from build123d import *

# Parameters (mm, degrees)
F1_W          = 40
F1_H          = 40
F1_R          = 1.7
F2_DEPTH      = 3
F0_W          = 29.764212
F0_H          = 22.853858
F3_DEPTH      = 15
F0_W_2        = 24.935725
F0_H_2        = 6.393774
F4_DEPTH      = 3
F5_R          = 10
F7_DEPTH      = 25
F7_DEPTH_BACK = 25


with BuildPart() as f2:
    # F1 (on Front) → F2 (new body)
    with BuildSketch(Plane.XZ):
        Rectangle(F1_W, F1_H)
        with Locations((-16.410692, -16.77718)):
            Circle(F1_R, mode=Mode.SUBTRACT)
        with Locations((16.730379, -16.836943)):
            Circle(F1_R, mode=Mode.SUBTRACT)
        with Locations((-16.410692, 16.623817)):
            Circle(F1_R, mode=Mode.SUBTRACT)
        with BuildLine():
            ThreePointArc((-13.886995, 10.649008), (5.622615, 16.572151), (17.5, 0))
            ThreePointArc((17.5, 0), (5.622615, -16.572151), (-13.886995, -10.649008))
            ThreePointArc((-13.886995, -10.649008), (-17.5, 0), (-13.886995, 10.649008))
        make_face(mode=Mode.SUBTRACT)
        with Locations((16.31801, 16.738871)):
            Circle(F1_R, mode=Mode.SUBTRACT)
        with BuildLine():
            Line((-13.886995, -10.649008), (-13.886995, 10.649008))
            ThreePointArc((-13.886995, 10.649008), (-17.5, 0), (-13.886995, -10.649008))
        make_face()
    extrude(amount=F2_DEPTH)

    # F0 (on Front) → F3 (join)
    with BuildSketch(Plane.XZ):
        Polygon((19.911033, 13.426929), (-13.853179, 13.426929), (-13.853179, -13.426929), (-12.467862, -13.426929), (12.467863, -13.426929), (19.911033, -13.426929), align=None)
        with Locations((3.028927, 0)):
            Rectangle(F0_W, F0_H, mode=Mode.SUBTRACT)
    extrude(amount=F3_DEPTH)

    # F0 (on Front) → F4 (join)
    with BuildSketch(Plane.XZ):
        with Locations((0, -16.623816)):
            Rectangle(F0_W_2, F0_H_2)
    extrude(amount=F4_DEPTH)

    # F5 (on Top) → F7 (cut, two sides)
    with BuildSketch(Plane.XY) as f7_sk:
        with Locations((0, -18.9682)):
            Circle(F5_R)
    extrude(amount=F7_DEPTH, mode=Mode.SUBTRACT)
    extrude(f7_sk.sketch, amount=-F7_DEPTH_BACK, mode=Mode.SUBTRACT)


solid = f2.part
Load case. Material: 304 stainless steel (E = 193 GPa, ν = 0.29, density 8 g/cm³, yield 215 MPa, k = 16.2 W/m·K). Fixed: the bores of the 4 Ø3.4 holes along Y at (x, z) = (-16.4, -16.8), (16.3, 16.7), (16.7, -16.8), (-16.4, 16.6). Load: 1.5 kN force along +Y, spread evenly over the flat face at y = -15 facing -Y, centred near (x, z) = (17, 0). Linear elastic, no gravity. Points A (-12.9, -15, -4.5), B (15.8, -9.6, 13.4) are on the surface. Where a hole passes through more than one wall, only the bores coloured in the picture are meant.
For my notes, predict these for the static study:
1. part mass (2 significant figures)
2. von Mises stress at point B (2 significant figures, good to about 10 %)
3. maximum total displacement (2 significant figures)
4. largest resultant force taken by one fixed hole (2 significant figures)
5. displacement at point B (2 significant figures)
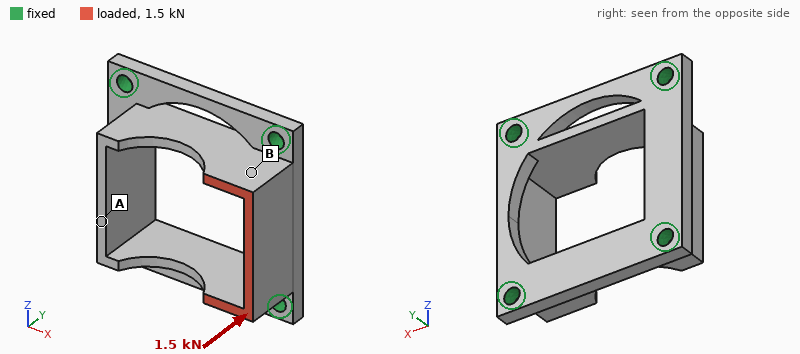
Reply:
40 g
23 MPa
8.6 µm
800 N
4.3 µm
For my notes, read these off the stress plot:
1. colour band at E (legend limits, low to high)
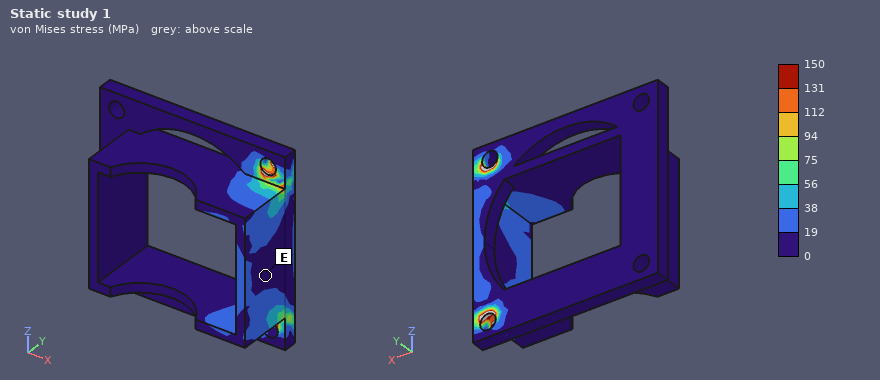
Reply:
0 to 19 MPa
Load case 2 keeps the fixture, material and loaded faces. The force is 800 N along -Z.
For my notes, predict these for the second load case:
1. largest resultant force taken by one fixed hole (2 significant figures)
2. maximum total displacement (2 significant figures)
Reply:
550 N
22 µm
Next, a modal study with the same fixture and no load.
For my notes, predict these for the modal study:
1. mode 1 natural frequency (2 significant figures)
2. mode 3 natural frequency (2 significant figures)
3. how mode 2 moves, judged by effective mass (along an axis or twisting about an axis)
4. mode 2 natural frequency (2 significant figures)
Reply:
11 kHz
14 kHz
along X
13 kHz
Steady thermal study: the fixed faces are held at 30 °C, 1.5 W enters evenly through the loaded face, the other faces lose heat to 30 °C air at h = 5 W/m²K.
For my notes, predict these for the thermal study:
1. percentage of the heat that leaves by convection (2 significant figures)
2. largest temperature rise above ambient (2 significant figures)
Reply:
7.7 %
20 K
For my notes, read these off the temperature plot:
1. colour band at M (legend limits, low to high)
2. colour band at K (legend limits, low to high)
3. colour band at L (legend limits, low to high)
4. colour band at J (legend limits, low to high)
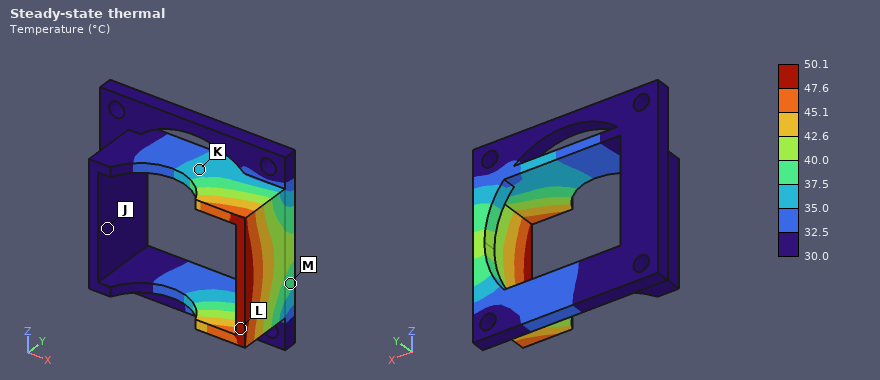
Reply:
37.5 to 40.0 °C
35.0 to 37.5 °C
47.6 to 50.1 °C
30.0 to 32.5 °C
